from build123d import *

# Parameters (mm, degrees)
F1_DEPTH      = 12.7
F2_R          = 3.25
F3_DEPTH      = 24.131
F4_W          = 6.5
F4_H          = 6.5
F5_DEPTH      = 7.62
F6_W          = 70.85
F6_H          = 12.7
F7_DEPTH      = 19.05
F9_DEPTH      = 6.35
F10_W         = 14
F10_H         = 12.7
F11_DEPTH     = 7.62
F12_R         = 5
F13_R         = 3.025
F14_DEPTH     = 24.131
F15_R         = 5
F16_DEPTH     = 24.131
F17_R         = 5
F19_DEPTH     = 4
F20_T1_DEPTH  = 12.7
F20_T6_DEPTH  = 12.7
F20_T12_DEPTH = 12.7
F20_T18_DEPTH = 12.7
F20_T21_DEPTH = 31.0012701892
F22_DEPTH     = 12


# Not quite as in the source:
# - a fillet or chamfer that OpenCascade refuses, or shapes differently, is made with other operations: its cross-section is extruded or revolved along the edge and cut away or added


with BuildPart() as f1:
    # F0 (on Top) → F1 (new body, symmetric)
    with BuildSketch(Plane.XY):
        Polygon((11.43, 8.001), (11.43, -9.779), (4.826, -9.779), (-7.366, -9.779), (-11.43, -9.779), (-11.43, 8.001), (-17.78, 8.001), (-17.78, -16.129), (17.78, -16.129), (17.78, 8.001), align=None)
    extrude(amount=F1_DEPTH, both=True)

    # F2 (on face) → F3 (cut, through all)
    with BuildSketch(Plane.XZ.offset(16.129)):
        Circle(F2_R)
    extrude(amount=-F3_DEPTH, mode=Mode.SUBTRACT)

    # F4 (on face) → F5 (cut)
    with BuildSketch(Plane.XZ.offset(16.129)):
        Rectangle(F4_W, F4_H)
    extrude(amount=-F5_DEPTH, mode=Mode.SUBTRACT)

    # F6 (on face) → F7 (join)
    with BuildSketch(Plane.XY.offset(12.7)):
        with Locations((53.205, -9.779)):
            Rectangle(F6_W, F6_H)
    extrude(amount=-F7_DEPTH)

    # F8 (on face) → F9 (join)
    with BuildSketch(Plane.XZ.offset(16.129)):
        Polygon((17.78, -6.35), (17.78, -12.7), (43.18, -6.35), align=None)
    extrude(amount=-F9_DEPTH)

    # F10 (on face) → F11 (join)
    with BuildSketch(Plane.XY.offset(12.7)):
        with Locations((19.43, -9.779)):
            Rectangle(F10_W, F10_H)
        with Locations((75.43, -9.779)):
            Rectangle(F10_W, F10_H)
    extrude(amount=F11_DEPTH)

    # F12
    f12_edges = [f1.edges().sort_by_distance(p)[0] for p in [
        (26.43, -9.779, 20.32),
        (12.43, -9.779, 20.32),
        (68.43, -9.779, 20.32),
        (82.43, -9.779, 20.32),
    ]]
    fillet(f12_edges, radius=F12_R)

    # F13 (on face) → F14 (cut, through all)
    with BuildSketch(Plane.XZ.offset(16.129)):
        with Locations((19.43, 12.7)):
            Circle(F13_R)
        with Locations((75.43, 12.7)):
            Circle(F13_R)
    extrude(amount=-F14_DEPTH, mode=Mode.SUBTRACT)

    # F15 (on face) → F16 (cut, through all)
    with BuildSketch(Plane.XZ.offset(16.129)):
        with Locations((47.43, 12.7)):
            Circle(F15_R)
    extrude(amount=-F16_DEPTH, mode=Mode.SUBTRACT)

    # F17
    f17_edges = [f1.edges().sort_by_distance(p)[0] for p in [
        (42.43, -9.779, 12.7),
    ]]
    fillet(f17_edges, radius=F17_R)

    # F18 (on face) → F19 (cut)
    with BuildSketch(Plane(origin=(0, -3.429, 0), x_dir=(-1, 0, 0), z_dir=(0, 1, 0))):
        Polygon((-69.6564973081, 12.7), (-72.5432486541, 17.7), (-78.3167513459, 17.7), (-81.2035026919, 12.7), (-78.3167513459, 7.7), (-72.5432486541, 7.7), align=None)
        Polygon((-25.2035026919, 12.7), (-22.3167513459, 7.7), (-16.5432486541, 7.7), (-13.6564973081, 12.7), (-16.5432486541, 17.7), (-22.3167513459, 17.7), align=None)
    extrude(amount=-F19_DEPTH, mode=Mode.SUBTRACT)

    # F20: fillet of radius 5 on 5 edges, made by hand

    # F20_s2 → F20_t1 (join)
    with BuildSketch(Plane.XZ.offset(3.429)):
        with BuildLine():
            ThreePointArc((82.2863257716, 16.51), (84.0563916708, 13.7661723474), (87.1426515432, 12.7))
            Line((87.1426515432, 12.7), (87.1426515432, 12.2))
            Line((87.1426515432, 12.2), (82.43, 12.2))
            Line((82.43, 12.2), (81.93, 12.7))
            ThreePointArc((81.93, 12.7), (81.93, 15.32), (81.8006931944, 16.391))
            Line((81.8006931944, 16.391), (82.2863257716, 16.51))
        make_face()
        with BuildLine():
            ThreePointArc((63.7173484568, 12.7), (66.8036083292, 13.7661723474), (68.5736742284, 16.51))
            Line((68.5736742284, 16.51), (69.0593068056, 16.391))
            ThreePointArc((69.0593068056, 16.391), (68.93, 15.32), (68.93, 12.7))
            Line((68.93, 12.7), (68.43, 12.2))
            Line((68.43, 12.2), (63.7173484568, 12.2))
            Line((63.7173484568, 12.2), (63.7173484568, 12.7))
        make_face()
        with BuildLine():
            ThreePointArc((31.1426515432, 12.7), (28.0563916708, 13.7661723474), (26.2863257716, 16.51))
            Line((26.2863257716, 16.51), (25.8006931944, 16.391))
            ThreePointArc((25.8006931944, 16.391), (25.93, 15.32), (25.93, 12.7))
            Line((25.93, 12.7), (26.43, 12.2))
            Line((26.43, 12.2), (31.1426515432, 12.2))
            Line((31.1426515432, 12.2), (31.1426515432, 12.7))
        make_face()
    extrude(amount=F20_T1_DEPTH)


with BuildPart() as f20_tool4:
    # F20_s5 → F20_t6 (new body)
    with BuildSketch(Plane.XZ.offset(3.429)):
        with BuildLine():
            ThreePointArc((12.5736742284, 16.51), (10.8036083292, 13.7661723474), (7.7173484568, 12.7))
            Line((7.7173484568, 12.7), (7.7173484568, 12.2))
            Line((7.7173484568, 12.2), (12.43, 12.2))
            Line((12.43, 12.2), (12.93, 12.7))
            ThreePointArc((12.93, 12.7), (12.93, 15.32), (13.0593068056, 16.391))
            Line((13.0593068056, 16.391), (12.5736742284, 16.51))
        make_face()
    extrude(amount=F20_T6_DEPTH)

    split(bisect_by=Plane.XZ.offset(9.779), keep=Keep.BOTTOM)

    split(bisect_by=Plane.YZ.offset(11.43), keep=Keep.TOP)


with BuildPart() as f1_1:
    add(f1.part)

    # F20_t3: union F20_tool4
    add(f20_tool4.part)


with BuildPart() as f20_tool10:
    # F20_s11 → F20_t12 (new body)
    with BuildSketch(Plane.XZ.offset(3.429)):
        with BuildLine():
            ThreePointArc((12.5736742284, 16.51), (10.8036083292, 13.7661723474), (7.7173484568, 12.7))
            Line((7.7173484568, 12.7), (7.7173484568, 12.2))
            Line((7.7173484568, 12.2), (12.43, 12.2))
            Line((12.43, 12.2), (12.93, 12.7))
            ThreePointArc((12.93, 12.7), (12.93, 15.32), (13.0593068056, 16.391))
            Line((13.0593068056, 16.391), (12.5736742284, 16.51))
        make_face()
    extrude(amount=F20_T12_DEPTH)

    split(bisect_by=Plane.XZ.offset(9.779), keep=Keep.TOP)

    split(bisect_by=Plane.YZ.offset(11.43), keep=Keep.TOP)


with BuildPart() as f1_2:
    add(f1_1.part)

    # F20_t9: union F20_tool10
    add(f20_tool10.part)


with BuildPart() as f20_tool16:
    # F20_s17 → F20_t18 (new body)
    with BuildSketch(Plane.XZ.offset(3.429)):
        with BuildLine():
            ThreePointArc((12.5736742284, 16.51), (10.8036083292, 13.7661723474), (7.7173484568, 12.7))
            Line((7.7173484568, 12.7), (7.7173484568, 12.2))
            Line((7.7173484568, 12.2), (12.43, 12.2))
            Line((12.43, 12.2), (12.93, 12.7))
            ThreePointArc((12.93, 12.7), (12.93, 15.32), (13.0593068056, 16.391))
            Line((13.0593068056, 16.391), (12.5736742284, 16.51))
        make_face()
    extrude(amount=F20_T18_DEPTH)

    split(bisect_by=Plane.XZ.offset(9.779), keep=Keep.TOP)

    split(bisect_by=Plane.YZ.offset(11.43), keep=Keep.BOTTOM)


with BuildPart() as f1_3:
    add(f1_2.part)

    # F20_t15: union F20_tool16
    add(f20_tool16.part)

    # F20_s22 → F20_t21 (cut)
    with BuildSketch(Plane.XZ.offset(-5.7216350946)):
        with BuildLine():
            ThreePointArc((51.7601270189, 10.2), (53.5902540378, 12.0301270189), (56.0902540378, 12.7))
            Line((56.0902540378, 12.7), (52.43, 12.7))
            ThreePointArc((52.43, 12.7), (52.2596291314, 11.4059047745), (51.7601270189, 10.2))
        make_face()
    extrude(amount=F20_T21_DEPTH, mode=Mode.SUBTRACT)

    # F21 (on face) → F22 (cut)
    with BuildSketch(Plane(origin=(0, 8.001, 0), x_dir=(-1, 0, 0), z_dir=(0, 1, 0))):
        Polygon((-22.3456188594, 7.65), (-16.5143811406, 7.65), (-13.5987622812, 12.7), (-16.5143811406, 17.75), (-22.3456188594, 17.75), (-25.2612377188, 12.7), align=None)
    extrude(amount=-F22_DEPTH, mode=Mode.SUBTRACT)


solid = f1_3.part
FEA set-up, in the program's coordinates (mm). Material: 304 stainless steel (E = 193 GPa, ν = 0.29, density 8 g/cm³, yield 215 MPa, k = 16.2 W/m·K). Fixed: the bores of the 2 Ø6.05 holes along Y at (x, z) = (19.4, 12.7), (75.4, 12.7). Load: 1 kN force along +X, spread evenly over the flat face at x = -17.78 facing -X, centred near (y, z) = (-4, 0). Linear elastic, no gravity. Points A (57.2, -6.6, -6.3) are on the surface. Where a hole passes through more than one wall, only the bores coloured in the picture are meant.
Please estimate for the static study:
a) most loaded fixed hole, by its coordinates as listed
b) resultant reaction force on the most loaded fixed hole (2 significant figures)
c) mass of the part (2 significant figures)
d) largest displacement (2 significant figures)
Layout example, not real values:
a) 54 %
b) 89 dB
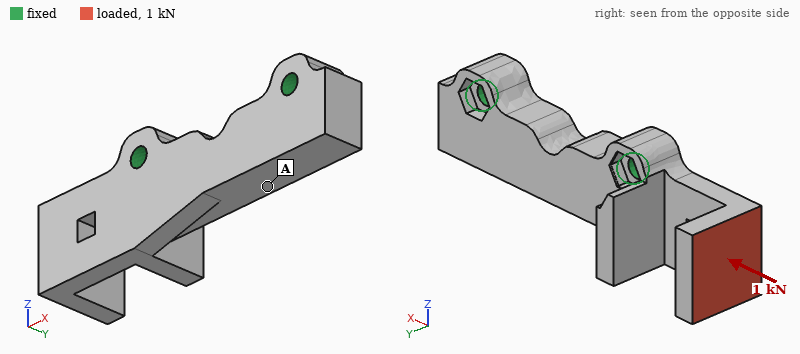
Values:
a) (19.4, 12.7)
b) 620 N
c) 240 g
d) 84 µm
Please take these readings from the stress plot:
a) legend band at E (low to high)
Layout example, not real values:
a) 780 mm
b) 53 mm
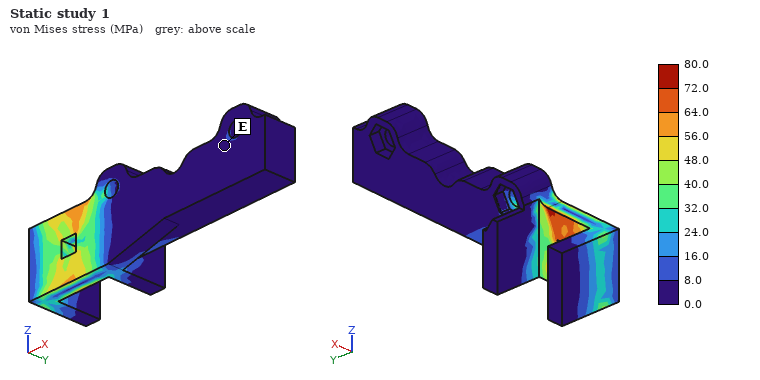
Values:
a) 0.0 to 8.0 MPa
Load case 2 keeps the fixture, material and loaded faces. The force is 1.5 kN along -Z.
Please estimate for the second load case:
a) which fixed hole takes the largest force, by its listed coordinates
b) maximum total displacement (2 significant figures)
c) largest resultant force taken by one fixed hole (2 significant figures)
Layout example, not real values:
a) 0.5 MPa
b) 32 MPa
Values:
a) (19.4, 12.7)
b) 93 µm
c) 2.7 kN
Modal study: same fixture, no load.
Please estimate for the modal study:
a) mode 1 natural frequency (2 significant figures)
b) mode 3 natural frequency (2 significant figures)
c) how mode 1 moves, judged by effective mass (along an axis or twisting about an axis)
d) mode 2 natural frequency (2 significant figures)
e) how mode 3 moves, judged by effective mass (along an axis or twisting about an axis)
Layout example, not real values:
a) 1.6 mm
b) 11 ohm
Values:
a) 2300 Hz
b) 7100 Hz
c) along Y
d) 4000 Hz
e) along Y
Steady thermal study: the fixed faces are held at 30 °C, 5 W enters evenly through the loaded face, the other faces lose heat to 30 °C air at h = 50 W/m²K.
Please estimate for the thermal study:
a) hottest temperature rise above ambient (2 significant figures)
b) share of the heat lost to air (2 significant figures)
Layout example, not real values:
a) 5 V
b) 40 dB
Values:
a) 40 K
b) 72 %
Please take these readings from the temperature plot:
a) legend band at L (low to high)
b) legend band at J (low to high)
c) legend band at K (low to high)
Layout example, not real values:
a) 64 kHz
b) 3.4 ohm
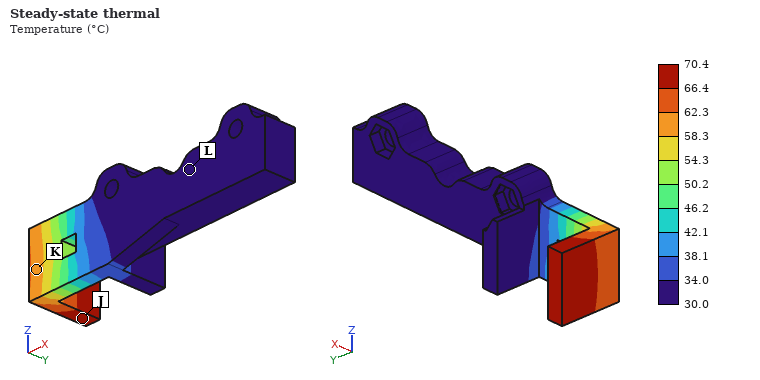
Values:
a) 30.0 to 34.0 °C
b) 66.4 to 70.4 °C
c) 58.3 to 62.3 °C
